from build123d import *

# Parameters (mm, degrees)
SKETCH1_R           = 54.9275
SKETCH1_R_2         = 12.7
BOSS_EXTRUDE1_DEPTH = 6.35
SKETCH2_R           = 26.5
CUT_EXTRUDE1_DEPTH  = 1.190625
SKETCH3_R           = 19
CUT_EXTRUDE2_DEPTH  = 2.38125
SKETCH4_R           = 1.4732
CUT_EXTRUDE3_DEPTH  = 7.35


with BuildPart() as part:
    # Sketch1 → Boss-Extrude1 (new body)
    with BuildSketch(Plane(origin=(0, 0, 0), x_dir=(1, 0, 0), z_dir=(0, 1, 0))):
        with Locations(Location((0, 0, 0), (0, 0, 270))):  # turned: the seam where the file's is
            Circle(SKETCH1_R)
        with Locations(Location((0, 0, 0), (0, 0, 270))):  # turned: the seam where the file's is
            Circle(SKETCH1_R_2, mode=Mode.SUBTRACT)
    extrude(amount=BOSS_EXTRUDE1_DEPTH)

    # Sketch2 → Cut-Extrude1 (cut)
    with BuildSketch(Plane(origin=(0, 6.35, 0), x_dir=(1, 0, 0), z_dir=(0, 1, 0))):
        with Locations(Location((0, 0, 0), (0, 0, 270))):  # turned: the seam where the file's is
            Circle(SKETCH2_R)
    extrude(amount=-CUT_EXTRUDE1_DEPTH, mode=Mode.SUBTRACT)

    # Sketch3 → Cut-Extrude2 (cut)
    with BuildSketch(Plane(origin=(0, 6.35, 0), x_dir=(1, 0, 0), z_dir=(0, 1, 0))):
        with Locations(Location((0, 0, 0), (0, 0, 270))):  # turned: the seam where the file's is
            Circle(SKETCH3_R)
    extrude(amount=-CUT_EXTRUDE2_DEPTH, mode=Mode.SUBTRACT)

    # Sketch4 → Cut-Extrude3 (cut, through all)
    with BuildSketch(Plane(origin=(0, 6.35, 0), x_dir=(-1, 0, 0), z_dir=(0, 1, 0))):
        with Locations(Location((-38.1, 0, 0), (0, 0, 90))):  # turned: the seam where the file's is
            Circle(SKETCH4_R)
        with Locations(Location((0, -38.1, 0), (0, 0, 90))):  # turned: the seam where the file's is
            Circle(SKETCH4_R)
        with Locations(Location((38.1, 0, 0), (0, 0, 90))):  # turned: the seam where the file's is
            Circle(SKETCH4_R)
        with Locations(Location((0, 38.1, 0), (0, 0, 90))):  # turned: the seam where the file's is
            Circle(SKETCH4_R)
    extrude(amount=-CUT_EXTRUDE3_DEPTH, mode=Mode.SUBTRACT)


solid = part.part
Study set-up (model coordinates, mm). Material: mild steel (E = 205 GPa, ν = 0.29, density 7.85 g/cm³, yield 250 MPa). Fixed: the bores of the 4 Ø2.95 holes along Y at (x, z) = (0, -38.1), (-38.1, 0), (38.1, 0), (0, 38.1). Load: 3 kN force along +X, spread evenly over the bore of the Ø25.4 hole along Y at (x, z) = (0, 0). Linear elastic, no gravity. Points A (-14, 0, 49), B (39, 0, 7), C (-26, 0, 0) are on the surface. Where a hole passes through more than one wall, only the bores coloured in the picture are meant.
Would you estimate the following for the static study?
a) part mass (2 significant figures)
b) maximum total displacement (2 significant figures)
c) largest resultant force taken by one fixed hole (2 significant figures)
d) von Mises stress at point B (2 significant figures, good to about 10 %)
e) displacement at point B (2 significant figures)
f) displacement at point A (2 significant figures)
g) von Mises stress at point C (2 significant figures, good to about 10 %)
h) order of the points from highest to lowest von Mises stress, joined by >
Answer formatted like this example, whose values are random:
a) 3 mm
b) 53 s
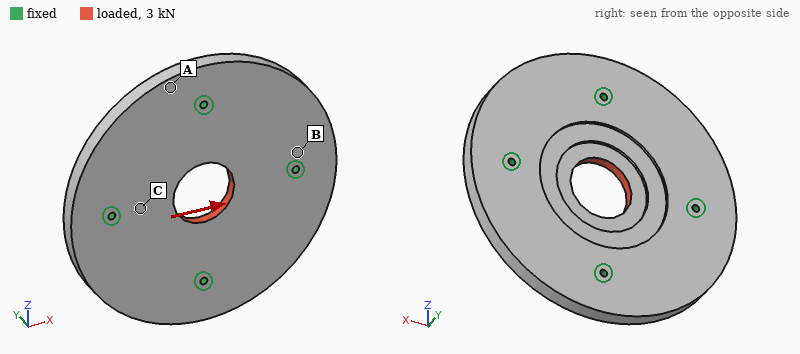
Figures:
a) 420 g
b) 1.6 µm
c) 890 N
d) 4.2 MPa
e) 0.37 µm
f) 0.28 µm
g) 10 MPa
h) C > B > A
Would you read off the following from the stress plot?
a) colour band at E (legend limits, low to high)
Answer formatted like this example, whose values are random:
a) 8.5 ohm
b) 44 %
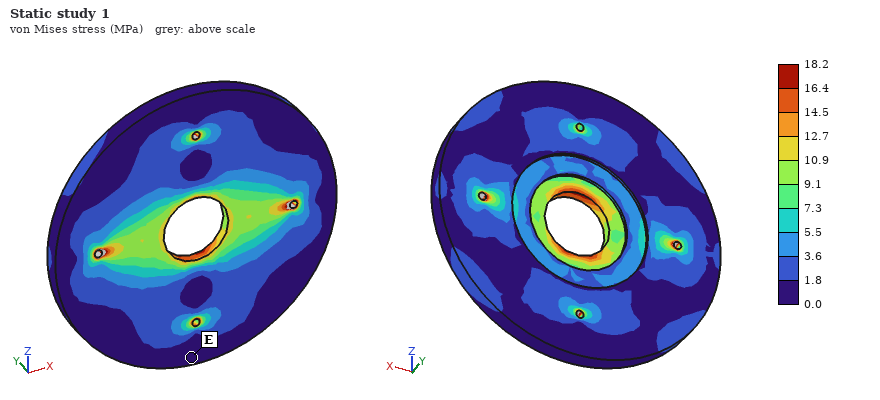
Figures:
a) 0.0 to 1.8 MPa
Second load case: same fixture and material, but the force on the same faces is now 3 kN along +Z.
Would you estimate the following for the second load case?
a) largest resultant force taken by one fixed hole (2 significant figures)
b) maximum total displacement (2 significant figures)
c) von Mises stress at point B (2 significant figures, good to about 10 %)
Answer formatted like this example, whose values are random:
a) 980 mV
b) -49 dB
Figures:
a) 890 N
b) 1.6 µm
c) 4.5 MPa
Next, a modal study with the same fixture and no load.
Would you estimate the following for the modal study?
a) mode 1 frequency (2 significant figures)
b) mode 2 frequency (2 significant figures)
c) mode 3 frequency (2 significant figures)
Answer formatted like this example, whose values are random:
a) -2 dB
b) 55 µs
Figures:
a) 4500 Hz
b) 5400 Hz
c) 5400 Hz
